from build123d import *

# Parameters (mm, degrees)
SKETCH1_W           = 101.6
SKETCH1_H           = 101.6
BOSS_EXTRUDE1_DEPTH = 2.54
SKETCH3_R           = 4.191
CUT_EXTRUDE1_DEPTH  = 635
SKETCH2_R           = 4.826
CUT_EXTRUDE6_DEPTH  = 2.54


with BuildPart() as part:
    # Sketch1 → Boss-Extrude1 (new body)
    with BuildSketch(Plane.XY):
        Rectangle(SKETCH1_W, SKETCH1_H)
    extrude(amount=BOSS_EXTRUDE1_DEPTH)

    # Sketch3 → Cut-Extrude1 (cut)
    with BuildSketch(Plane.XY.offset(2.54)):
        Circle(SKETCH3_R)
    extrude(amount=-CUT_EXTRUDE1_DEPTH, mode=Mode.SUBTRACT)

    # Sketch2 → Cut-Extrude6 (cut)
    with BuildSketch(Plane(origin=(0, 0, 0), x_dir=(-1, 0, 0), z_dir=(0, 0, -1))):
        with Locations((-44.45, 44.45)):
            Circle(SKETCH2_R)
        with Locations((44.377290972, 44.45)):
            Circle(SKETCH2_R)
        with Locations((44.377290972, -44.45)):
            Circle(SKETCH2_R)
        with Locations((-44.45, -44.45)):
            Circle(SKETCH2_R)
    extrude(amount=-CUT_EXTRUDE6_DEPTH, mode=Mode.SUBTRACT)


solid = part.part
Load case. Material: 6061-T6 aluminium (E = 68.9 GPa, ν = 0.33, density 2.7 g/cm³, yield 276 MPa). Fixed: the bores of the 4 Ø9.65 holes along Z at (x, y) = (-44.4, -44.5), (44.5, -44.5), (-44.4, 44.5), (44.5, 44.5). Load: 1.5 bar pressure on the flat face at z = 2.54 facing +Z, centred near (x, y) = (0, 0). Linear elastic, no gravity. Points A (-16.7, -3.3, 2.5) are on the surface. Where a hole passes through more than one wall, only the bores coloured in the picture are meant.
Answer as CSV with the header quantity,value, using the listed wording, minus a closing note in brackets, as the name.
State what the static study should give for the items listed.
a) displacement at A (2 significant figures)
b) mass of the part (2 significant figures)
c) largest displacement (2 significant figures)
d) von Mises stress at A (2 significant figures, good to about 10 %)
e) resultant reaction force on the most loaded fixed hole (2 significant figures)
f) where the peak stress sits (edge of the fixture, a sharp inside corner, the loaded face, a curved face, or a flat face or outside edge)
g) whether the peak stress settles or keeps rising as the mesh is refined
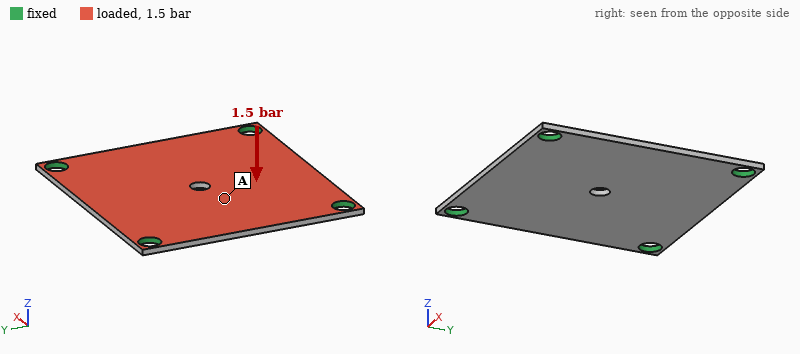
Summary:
quantity,value
displacement at A,0.48 mm
mass of the part,68 g
largest displacement,0.55 mm
von Mises stress at A,49 MPa
resultant reaction force on the most loaded fixed hole,370 N
where the peak stress sits,edge of the fixture
whether the peak stress settles or keeps rising as the mesh is refined,keeps rising
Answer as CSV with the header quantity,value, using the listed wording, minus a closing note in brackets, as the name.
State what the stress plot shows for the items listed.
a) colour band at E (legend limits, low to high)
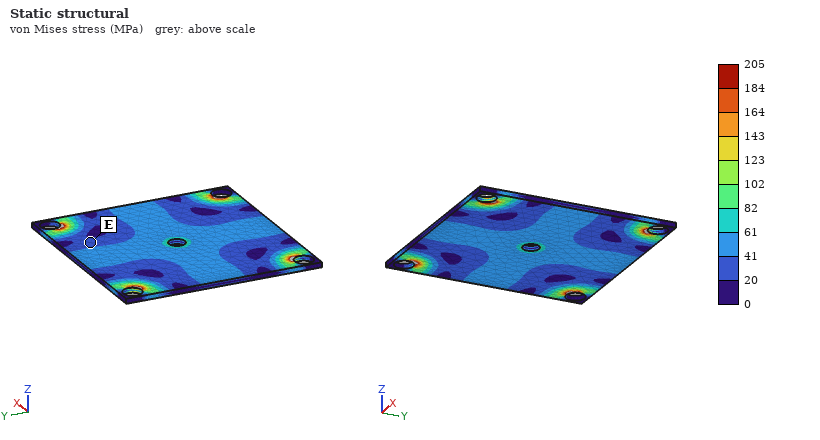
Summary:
quantity,value
colour band at E,20 to 41 MPa
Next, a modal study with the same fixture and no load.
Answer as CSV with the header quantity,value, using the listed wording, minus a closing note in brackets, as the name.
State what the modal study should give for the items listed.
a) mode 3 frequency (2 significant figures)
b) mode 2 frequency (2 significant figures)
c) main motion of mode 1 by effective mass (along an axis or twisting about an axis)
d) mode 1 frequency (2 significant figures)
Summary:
quantity,value
mode 3 frequency,2100 Hz
mode 2 frequency,2100 Hz
main motion of mode 1 by effective mass,along Z
mode 1 frequency,1300 Hz
